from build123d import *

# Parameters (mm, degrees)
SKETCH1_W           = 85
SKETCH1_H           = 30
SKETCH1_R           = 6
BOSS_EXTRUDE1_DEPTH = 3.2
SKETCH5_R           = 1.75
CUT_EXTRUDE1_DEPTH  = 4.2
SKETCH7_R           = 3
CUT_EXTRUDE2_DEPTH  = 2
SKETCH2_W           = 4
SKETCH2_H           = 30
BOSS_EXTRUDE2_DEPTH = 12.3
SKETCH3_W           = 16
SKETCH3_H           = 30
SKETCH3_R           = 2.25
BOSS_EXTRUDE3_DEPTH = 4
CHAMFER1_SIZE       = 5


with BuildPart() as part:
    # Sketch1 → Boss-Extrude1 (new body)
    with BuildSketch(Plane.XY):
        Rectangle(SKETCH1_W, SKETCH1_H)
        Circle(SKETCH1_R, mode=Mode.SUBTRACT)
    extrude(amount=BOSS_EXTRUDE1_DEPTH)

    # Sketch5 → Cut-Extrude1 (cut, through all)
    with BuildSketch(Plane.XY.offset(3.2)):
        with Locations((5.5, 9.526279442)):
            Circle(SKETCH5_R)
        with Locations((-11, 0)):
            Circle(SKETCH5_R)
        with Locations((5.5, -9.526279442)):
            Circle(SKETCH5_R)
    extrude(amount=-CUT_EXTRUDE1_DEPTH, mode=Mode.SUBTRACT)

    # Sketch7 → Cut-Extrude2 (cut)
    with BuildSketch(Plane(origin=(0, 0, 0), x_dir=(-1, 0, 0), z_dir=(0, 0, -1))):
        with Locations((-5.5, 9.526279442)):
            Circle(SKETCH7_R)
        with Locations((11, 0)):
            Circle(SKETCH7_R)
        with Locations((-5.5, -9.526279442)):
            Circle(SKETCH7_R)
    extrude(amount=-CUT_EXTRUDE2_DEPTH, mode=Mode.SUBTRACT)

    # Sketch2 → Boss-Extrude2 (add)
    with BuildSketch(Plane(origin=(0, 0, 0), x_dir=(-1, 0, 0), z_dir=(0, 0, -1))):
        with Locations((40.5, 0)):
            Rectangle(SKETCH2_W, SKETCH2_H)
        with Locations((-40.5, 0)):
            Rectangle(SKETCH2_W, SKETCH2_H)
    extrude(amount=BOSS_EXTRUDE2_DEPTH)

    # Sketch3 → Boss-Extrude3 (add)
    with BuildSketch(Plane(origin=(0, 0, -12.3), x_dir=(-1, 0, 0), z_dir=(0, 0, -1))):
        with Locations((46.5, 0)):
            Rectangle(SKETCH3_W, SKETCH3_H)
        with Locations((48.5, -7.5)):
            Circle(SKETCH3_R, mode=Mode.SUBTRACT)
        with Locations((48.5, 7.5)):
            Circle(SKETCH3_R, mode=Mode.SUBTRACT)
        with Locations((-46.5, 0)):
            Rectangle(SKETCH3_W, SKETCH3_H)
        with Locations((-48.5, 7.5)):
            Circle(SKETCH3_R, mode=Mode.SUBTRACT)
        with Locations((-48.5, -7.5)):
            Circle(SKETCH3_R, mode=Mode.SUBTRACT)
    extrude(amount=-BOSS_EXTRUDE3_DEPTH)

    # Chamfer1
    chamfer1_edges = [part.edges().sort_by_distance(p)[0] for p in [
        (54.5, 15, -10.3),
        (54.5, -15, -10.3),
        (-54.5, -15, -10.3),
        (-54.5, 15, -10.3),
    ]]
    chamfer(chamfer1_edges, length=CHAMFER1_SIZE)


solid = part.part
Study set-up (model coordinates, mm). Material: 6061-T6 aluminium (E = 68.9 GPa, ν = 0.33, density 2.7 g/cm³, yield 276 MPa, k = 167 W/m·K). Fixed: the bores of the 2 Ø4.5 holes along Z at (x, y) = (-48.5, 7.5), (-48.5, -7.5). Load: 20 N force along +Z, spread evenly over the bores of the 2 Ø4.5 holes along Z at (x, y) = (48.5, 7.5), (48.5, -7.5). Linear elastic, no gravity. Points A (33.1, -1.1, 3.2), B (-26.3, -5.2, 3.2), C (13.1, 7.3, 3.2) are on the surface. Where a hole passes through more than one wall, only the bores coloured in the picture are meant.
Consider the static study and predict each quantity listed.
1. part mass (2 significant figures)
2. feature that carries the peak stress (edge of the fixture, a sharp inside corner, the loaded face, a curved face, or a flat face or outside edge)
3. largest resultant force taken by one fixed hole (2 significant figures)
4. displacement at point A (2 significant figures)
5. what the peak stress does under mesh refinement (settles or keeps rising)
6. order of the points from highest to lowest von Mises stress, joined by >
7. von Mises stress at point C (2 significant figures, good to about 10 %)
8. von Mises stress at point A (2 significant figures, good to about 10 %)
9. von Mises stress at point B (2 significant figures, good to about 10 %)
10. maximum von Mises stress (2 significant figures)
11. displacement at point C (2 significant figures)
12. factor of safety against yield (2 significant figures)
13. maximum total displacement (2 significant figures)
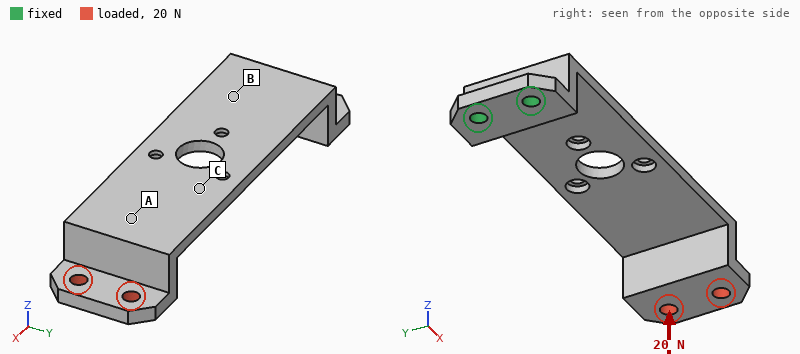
35 g
a curved face
10 N
0.87 mm
settles
B > C > A
14 MPa
5.9 MPa
27 MPa
69 MPa
0.52 mm
4.0
1.3 mm
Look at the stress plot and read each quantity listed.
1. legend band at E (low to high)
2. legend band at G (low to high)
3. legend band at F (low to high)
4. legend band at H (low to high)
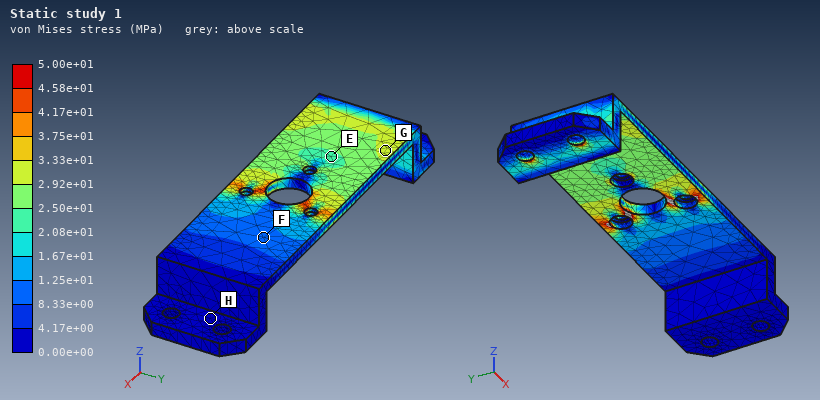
2.08e+01 to 2.50e+01 MPa
2.92e+01 to 3.33e+01 MPa
8.33e+00 to 1.25e+01 MPa
0.00e+00 to 4.17e+00 MPa
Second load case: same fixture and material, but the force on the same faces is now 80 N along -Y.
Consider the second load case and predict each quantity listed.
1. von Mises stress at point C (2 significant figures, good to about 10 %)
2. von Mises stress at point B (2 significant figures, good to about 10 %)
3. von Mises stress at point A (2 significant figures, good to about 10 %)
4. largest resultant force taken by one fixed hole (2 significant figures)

19 MPa
20 MPa
9.2 MPa
420 N
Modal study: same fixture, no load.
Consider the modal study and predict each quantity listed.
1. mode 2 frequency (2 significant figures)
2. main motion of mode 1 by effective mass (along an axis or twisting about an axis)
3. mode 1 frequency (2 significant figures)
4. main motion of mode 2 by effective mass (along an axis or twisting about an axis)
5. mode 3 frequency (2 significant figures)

680 Hz
along Z
200 Hz
along Y
1200 Hz
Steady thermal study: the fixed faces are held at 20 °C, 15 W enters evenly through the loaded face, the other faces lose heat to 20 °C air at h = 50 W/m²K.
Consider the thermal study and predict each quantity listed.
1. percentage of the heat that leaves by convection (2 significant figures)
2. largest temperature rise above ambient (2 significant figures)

69 %
56 K
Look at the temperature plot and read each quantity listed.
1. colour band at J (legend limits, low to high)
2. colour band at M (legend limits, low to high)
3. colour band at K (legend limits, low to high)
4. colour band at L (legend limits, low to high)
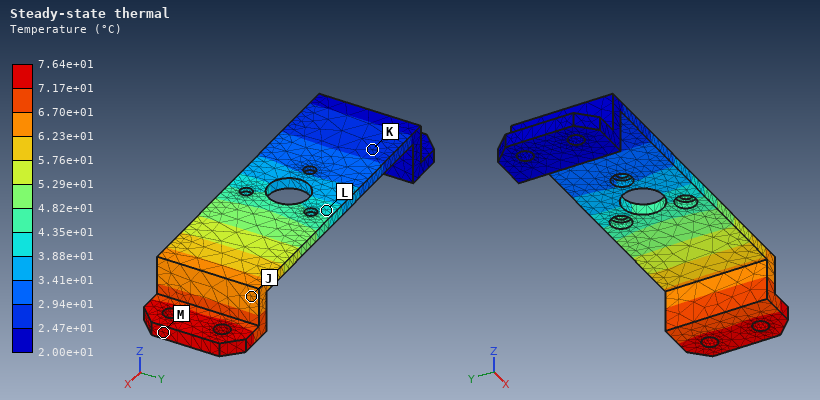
6.23e+01 to 6.70e+01 °C
7.17e+01 to 7.64e+01 °C
2.47e+01 to 2.94e+01 °C
3.88e+01 to 4.35e+01 °C
